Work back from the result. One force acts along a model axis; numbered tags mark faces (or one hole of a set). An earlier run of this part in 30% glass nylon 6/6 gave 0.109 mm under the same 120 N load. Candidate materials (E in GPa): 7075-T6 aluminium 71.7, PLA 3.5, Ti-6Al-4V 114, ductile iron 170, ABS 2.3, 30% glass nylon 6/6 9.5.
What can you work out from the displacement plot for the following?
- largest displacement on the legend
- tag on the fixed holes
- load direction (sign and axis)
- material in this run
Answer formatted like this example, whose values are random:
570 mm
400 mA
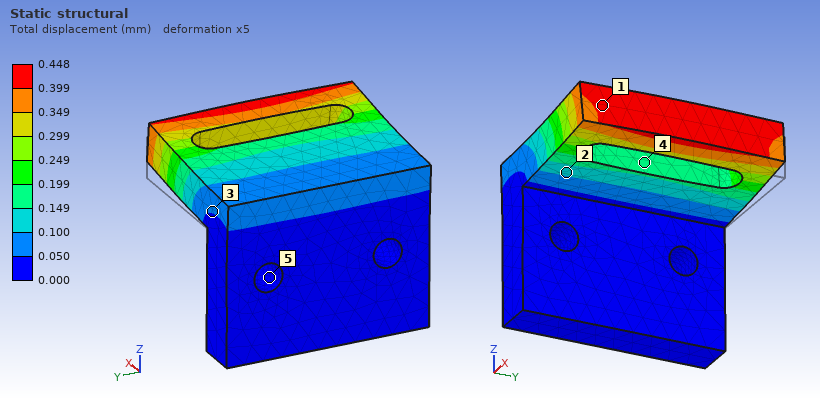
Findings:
0.448 mm
5
+Z
ABS
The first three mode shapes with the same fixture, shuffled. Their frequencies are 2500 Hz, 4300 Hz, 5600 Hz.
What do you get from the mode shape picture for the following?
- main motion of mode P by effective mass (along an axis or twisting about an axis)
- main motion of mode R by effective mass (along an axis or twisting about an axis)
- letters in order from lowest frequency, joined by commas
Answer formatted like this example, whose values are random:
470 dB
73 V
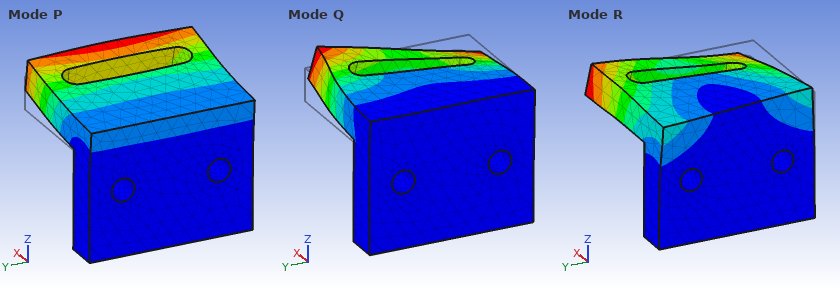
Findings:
along Z
along Y
P, R, Q
